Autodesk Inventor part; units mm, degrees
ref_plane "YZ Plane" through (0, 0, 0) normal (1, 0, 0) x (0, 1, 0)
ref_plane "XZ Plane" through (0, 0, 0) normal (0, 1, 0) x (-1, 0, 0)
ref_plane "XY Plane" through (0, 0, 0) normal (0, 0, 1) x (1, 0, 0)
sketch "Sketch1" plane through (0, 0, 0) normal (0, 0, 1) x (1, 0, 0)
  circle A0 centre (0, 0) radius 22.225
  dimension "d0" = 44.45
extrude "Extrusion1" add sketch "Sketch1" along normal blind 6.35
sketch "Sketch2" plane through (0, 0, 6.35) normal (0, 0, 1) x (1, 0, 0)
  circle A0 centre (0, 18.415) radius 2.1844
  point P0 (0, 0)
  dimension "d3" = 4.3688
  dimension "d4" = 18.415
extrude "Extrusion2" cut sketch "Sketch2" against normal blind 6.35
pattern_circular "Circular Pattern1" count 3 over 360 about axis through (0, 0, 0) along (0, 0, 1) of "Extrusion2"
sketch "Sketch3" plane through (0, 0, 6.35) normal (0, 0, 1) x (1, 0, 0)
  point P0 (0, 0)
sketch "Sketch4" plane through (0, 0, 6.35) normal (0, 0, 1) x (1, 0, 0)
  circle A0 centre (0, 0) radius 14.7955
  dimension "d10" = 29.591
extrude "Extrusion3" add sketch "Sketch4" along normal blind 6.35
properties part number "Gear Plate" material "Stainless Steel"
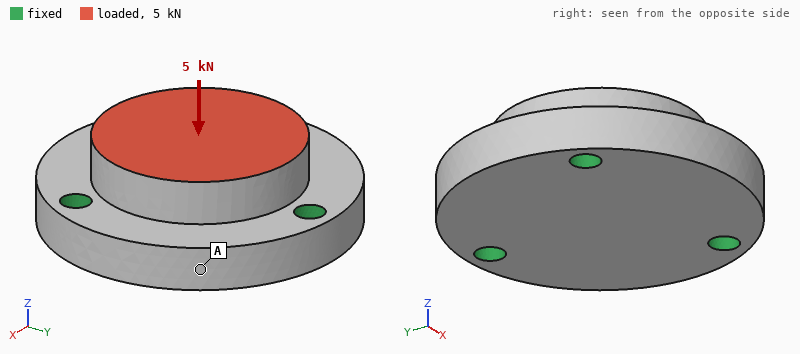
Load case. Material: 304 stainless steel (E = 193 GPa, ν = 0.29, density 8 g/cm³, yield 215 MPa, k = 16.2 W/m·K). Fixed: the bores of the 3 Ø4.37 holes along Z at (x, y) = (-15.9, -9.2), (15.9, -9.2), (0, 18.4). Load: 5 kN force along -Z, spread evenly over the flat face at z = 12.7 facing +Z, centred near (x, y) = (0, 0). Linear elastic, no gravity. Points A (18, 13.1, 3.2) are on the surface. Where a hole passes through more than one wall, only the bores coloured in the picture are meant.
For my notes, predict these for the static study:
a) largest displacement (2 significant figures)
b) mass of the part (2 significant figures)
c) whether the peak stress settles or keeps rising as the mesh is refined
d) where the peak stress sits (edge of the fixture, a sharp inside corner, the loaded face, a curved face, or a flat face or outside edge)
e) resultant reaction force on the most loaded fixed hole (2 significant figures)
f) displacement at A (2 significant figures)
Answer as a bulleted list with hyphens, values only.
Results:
- 3.1 µm
- 110 g
- keeps rising
- edge of the fixture
- 1.8 kN
- 2.4 µm
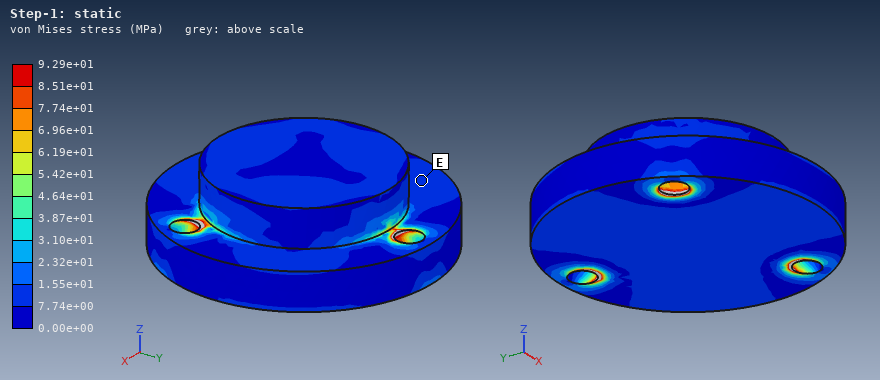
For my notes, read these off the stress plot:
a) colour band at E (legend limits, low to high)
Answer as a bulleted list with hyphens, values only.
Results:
- 7.74e+00 to 1.55e+01 MPa
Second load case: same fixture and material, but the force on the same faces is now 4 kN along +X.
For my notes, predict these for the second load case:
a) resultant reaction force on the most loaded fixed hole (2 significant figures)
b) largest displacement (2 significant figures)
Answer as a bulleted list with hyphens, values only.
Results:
- 1.9 kN
- 3.7 µm
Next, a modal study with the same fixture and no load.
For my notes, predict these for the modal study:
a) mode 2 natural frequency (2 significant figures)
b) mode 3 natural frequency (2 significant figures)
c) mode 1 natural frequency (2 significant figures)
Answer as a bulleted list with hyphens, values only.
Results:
- 23 kHz
- 23 kHz
- 22 kHz
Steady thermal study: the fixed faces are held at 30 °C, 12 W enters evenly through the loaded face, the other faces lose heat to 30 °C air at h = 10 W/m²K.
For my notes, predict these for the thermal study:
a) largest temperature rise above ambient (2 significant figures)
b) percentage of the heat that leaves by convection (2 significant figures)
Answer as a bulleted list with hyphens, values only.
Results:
- 24 K
- 3.5 %
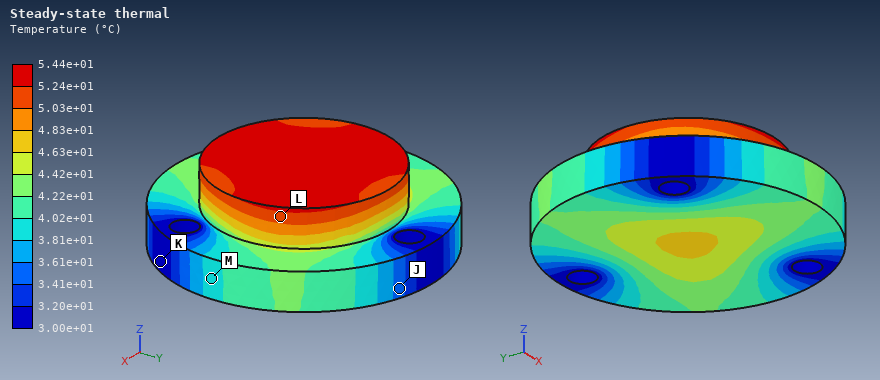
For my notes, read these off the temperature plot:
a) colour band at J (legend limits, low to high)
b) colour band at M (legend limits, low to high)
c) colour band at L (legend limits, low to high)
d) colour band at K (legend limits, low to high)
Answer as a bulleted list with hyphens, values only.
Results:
- 3.41e+01 to 3.61e+01 °C
- 3.81e+01 to 4.02e+01 °C
- 5.03e+01 to 5.24e+01 °C
- 3.00e+01 to 3.20e+01 °C
